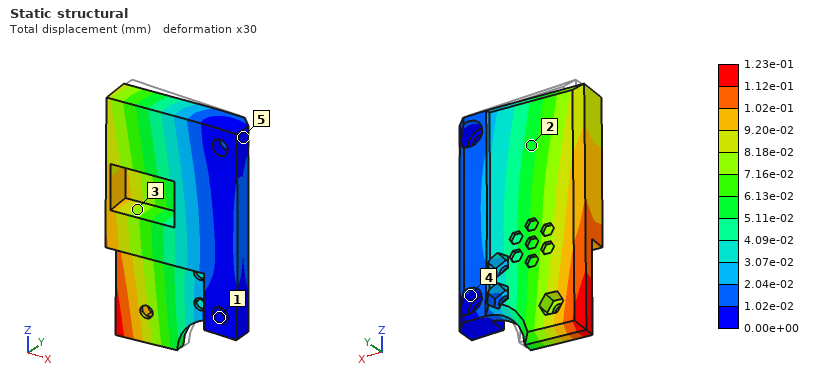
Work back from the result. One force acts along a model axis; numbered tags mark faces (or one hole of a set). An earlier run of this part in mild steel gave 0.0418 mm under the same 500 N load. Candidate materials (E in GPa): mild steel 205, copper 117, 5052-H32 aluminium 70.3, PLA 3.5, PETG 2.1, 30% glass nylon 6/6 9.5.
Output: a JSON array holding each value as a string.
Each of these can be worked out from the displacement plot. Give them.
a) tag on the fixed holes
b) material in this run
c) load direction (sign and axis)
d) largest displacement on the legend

["1", "5052-H32 aluminium", "-Y", "1.23e-01 mm"]
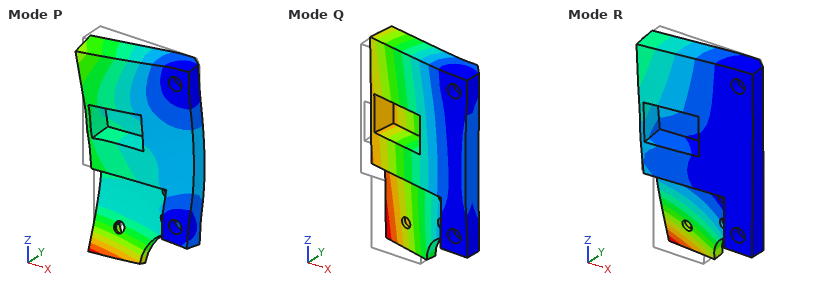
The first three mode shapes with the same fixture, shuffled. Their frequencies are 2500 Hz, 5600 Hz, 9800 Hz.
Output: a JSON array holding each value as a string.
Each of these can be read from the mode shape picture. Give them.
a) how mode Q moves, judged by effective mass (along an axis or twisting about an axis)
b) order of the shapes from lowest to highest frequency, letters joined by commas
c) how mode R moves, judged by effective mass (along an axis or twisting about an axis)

["along Y", "Q, R, P", "twisting about X"]
